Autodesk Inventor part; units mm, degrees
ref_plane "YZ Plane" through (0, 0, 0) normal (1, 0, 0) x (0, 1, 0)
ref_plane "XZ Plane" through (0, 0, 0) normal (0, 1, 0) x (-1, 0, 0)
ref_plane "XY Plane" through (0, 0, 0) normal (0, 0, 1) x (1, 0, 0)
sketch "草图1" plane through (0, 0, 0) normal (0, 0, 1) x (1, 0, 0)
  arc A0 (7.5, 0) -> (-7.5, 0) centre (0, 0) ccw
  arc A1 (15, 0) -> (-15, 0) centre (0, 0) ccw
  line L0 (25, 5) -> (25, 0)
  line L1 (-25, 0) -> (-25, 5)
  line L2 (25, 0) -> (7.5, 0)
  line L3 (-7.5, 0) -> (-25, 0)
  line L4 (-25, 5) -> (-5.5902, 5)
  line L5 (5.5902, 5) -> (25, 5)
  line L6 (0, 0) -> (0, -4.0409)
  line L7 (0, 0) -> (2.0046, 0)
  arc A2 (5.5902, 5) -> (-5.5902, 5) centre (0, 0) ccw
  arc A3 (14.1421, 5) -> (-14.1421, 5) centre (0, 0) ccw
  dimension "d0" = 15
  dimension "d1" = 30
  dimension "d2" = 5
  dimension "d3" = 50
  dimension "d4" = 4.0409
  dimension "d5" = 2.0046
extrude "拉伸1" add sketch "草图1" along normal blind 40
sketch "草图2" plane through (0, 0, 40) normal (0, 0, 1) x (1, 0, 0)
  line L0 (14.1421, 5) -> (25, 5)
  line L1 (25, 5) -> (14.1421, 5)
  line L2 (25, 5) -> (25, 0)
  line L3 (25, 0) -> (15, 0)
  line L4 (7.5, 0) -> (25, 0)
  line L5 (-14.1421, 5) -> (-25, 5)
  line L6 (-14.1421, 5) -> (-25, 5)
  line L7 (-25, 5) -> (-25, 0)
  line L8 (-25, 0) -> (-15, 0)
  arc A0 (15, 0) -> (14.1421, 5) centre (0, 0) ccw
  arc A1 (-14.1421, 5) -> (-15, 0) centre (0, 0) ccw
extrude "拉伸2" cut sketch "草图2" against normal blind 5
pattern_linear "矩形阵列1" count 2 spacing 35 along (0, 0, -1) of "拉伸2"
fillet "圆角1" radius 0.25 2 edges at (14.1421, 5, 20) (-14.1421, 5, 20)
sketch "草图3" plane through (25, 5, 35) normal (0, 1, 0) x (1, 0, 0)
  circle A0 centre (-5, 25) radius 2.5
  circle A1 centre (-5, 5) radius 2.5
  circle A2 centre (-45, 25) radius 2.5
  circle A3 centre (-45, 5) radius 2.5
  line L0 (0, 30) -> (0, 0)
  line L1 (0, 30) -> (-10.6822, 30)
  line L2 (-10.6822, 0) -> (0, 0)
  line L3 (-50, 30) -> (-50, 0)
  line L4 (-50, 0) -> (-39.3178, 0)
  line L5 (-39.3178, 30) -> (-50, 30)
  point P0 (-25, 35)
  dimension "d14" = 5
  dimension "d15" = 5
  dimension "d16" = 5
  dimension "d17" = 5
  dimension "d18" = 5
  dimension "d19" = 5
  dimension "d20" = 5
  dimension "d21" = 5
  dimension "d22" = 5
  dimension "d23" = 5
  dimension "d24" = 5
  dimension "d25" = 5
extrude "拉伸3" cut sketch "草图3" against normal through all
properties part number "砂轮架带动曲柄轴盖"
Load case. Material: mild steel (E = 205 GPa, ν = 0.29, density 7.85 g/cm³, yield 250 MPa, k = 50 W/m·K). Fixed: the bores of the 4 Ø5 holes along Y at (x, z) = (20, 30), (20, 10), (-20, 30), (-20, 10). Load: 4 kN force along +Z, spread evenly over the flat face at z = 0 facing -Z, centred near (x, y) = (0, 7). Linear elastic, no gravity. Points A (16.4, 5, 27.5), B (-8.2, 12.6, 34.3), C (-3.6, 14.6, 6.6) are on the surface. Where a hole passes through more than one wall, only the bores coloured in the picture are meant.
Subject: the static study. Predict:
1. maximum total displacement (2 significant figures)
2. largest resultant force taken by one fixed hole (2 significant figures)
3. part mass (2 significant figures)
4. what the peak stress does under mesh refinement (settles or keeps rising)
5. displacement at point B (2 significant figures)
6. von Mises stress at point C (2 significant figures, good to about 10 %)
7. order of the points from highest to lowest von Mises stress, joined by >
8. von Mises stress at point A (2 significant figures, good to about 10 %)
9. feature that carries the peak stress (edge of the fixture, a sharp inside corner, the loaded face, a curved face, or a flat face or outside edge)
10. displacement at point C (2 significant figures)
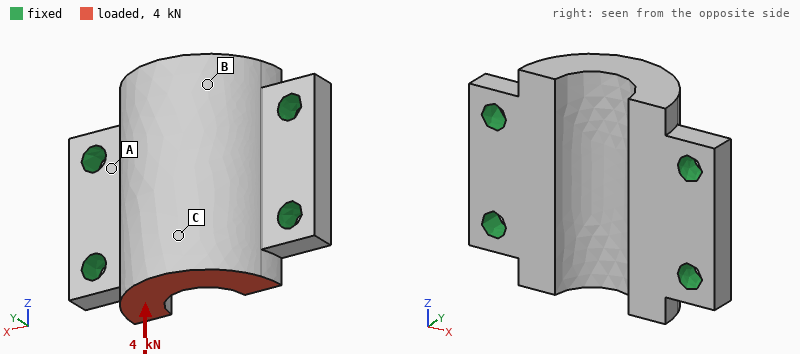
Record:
7.3 µm
1.4 kN
100 g
keeps rising
4.0 µm
19 MPa
A > C > B
39 MPa
edge of the fixture
5.8 µm
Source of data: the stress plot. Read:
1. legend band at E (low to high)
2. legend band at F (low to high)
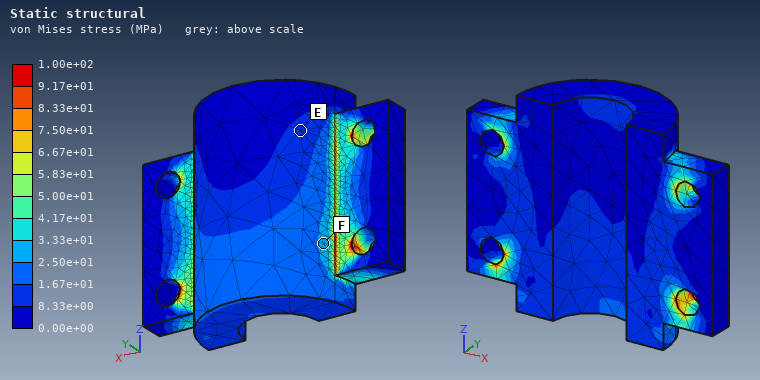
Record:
8.33e+00 to 1.67e+01 MPa
2.50e+01 to 3.33e+01 MPa
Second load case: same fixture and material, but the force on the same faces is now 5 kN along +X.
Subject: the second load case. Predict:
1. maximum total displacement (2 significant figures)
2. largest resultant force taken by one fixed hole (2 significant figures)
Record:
9.3 µm
2.5 kN
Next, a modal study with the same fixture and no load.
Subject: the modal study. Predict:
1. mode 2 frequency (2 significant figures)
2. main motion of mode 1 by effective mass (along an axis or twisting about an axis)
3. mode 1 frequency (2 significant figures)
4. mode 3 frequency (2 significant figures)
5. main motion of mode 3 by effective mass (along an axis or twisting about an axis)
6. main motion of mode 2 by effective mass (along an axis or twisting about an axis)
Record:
19 kHz
along Z
15 kHz
30 kHz
along Z
along Y
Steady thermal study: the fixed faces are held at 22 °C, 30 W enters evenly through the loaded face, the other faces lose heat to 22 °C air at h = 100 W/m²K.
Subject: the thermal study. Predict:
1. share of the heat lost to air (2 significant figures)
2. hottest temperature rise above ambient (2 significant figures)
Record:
19 %
44 K
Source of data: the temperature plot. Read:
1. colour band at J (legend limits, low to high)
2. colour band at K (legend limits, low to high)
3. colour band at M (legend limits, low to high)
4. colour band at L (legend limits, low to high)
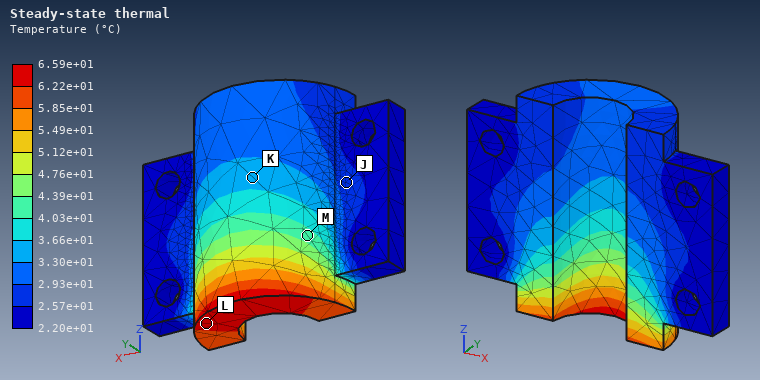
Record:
2.57e+01 to 2.93e+01 °C
3.30e+01 to 3.66e+01 °C
4.03e+01 to 4.39e+01 °C
6.22e+01 to 6.59e+01 °C
